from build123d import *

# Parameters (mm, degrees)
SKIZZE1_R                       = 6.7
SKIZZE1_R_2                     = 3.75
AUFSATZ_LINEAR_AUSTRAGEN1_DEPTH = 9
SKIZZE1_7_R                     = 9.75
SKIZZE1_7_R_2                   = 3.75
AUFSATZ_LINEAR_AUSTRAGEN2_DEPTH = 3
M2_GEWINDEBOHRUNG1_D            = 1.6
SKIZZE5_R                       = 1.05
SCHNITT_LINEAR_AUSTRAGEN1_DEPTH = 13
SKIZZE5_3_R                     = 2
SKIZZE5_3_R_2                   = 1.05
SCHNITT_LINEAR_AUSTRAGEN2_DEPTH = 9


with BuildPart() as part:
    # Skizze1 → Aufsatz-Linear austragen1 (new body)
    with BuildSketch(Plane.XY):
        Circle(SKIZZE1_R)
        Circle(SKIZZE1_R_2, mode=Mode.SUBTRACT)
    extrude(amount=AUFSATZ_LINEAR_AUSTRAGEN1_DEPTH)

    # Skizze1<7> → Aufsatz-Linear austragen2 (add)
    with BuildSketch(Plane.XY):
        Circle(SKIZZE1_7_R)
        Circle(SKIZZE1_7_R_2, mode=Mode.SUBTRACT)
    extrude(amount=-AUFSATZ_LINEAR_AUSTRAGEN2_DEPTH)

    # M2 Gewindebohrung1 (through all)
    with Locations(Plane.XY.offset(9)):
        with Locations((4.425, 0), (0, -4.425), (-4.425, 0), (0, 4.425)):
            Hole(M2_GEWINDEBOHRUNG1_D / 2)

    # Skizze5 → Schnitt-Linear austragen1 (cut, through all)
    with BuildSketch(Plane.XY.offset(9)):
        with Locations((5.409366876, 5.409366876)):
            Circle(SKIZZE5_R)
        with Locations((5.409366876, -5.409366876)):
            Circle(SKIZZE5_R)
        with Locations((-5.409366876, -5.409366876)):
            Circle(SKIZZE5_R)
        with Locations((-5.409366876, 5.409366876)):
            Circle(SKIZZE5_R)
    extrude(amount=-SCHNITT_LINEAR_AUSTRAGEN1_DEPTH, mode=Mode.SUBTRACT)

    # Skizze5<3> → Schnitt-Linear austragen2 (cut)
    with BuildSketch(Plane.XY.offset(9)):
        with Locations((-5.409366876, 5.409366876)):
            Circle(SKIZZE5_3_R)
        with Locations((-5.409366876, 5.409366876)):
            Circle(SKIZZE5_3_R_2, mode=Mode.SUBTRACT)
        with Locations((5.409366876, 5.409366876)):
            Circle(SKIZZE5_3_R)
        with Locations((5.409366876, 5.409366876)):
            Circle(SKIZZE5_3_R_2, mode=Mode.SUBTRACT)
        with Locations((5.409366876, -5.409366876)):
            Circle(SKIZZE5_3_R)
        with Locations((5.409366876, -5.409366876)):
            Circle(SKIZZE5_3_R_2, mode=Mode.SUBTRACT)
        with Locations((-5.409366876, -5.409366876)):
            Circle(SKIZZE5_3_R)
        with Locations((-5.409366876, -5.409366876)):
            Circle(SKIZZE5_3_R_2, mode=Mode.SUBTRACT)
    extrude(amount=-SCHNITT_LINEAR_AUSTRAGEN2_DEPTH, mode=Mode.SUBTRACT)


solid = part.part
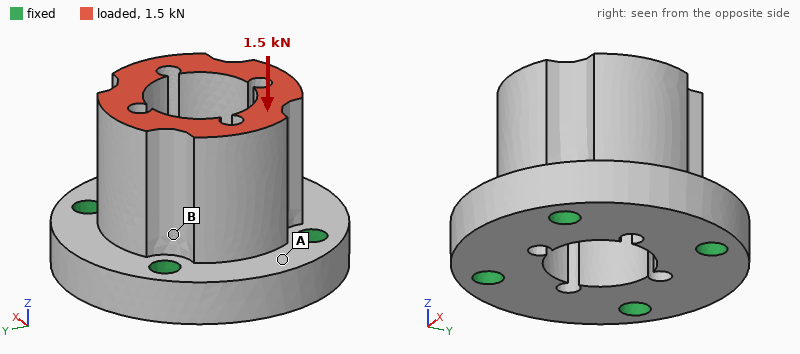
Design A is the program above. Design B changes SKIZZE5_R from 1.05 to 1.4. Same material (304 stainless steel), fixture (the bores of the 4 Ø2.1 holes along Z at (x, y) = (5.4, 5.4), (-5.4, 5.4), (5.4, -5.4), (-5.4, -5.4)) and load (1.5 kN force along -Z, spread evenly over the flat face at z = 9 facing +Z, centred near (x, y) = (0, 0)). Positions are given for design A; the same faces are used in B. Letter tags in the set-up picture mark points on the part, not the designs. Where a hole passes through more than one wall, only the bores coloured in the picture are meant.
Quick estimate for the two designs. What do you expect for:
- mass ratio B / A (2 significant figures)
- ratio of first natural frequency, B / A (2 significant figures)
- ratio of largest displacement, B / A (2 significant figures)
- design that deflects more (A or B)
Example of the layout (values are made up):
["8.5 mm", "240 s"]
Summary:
["0.98", "1.1", "0.87", "A"]
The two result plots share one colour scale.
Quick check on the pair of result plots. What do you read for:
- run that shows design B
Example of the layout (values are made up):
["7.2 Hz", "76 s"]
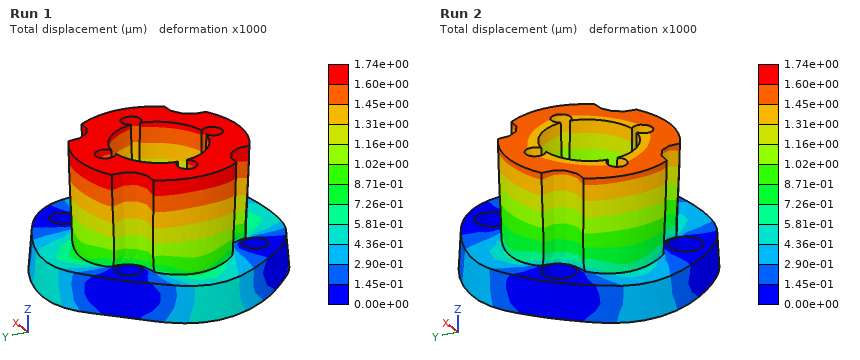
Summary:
["Run 2"]
